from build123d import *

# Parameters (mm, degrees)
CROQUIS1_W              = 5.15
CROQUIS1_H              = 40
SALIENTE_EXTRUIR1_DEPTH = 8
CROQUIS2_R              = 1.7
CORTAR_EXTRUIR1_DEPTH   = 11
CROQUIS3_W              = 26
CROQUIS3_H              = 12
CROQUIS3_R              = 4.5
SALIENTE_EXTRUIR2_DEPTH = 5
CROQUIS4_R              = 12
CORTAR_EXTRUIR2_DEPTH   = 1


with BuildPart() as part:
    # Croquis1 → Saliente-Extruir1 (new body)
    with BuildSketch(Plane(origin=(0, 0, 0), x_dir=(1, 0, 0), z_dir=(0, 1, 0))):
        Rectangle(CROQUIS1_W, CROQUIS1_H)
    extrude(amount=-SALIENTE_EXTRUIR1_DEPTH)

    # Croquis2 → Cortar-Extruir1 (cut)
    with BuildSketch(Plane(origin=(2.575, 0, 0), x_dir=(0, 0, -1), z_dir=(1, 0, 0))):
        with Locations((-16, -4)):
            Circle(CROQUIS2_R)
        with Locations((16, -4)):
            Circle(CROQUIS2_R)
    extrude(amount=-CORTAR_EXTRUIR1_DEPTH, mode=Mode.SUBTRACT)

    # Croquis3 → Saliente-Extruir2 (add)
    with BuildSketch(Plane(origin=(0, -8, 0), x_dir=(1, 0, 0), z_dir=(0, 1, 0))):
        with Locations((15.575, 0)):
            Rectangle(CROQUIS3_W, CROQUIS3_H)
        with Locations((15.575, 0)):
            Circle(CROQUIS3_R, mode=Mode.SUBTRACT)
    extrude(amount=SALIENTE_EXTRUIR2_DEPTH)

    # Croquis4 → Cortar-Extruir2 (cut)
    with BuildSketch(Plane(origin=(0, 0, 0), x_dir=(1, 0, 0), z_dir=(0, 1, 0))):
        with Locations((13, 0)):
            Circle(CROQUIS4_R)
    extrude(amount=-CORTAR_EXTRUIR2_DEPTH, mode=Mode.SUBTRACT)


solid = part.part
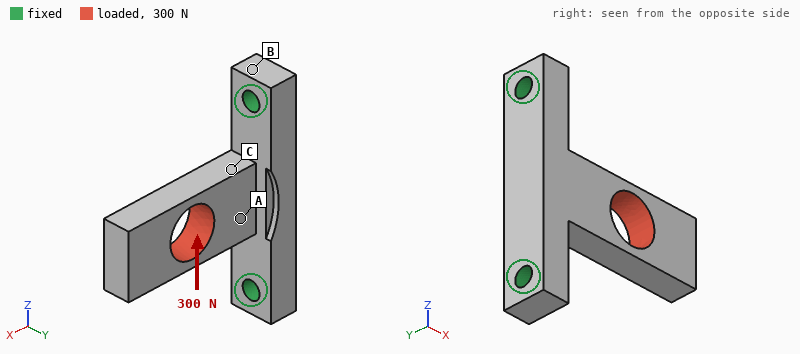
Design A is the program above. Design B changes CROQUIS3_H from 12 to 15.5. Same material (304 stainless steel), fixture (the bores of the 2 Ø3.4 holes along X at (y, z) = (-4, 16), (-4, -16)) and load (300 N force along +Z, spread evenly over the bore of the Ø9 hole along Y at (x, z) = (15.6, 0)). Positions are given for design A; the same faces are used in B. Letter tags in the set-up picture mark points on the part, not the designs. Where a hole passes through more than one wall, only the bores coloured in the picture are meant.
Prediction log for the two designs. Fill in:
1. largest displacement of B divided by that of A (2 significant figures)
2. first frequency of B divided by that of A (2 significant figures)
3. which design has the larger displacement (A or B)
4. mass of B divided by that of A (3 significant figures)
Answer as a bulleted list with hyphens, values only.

- 0.49
- 0.99
- A
- 1.16
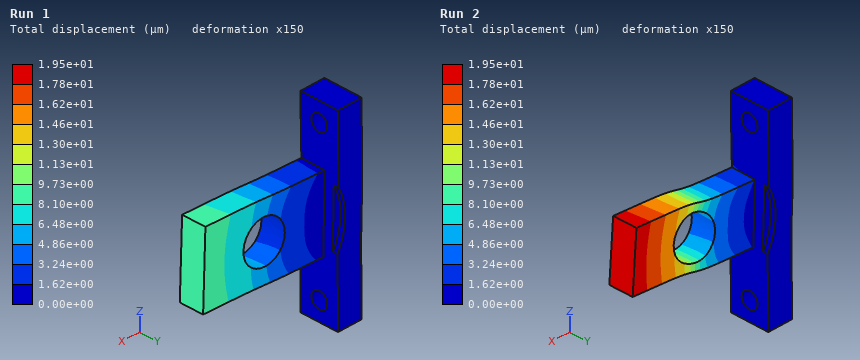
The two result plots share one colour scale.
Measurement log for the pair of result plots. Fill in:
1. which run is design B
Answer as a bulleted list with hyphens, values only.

- Run 1
